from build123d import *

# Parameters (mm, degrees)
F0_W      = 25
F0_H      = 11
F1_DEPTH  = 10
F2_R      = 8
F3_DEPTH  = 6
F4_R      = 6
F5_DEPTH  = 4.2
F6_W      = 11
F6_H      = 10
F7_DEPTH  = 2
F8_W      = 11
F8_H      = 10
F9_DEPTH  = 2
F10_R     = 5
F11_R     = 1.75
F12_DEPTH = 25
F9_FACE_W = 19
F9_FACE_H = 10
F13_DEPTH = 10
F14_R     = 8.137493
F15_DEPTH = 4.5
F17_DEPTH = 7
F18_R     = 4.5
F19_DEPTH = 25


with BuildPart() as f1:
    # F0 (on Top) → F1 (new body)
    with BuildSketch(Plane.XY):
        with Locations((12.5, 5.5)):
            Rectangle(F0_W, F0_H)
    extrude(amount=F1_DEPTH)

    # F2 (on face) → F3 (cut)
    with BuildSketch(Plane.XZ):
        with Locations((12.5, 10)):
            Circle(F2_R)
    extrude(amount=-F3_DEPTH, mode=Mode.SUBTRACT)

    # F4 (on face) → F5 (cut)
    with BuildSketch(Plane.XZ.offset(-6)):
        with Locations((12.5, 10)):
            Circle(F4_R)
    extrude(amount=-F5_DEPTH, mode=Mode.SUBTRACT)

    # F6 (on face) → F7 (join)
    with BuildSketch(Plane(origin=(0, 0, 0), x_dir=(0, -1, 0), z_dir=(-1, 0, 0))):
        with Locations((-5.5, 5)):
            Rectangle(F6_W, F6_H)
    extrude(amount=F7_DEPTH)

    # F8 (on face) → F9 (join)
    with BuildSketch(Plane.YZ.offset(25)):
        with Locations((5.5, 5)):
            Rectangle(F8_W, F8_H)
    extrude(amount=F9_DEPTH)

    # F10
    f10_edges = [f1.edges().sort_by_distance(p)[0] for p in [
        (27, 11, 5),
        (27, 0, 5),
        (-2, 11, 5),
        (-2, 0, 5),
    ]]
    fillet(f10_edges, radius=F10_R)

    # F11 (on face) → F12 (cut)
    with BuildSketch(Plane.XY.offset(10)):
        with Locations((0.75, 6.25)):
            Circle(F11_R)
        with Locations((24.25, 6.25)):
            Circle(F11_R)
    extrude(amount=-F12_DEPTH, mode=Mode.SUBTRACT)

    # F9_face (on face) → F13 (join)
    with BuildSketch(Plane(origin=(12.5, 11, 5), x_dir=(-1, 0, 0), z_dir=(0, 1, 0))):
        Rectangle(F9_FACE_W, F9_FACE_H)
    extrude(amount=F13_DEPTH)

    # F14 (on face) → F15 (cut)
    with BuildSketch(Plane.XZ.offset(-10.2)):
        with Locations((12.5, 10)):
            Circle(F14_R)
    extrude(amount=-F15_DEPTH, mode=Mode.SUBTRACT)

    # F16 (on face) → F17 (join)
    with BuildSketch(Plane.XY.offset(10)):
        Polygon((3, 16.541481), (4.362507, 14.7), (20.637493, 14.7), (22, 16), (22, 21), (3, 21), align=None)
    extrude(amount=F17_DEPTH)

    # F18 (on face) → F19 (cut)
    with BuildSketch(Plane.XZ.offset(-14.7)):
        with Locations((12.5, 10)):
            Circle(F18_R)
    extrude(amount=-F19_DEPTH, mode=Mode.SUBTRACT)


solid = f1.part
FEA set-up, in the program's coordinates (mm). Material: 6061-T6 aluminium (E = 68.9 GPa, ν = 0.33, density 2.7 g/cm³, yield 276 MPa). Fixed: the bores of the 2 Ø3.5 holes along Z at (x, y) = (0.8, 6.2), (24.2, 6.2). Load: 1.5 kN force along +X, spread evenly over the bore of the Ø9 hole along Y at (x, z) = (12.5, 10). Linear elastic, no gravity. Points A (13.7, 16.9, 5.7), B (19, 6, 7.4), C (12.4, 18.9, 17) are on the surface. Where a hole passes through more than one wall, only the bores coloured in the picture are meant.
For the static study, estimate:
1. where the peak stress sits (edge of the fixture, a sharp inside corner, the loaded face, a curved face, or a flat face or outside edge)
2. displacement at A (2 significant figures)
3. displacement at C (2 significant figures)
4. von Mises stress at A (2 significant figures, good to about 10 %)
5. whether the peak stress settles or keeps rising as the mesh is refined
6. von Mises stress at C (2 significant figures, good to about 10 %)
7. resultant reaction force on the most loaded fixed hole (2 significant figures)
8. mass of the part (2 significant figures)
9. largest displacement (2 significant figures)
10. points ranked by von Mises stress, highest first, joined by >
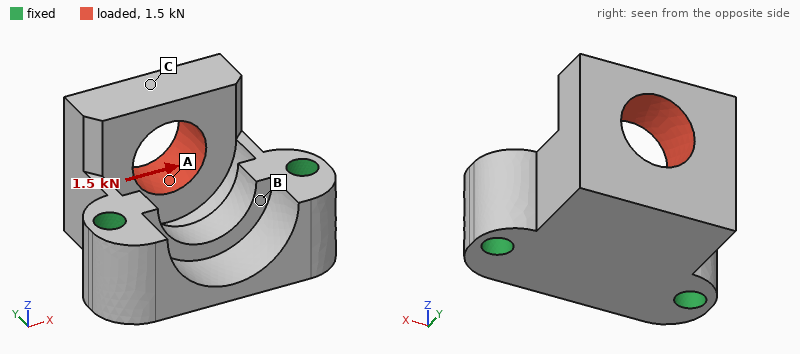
a sharp inside corner
17 µm
47 µm
63 MPa
keeps rising
26 MPa
1.1 kN
10 g
57 µm
A > C > B
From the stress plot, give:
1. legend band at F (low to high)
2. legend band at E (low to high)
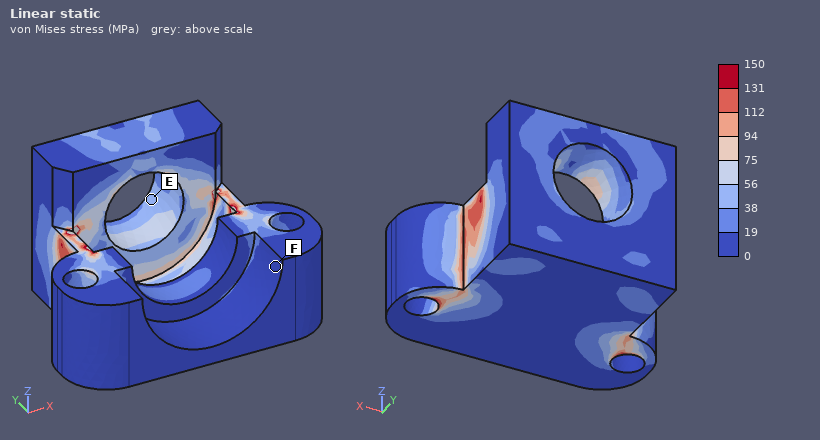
0 to 19 MPa
38 to 56 MPa
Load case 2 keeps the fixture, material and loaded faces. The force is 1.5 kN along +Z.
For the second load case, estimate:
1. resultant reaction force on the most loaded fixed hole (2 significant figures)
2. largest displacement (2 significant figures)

750 N
55 µm
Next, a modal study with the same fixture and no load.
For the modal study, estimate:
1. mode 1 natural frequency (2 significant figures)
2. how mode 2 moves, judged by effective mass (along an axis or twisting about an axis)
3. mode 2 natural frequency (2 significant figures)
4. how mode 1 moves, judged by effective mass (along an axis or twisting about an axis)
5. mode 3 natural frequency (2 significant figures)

13 kHz
along X
16 kHz
along Z
26 kHz
